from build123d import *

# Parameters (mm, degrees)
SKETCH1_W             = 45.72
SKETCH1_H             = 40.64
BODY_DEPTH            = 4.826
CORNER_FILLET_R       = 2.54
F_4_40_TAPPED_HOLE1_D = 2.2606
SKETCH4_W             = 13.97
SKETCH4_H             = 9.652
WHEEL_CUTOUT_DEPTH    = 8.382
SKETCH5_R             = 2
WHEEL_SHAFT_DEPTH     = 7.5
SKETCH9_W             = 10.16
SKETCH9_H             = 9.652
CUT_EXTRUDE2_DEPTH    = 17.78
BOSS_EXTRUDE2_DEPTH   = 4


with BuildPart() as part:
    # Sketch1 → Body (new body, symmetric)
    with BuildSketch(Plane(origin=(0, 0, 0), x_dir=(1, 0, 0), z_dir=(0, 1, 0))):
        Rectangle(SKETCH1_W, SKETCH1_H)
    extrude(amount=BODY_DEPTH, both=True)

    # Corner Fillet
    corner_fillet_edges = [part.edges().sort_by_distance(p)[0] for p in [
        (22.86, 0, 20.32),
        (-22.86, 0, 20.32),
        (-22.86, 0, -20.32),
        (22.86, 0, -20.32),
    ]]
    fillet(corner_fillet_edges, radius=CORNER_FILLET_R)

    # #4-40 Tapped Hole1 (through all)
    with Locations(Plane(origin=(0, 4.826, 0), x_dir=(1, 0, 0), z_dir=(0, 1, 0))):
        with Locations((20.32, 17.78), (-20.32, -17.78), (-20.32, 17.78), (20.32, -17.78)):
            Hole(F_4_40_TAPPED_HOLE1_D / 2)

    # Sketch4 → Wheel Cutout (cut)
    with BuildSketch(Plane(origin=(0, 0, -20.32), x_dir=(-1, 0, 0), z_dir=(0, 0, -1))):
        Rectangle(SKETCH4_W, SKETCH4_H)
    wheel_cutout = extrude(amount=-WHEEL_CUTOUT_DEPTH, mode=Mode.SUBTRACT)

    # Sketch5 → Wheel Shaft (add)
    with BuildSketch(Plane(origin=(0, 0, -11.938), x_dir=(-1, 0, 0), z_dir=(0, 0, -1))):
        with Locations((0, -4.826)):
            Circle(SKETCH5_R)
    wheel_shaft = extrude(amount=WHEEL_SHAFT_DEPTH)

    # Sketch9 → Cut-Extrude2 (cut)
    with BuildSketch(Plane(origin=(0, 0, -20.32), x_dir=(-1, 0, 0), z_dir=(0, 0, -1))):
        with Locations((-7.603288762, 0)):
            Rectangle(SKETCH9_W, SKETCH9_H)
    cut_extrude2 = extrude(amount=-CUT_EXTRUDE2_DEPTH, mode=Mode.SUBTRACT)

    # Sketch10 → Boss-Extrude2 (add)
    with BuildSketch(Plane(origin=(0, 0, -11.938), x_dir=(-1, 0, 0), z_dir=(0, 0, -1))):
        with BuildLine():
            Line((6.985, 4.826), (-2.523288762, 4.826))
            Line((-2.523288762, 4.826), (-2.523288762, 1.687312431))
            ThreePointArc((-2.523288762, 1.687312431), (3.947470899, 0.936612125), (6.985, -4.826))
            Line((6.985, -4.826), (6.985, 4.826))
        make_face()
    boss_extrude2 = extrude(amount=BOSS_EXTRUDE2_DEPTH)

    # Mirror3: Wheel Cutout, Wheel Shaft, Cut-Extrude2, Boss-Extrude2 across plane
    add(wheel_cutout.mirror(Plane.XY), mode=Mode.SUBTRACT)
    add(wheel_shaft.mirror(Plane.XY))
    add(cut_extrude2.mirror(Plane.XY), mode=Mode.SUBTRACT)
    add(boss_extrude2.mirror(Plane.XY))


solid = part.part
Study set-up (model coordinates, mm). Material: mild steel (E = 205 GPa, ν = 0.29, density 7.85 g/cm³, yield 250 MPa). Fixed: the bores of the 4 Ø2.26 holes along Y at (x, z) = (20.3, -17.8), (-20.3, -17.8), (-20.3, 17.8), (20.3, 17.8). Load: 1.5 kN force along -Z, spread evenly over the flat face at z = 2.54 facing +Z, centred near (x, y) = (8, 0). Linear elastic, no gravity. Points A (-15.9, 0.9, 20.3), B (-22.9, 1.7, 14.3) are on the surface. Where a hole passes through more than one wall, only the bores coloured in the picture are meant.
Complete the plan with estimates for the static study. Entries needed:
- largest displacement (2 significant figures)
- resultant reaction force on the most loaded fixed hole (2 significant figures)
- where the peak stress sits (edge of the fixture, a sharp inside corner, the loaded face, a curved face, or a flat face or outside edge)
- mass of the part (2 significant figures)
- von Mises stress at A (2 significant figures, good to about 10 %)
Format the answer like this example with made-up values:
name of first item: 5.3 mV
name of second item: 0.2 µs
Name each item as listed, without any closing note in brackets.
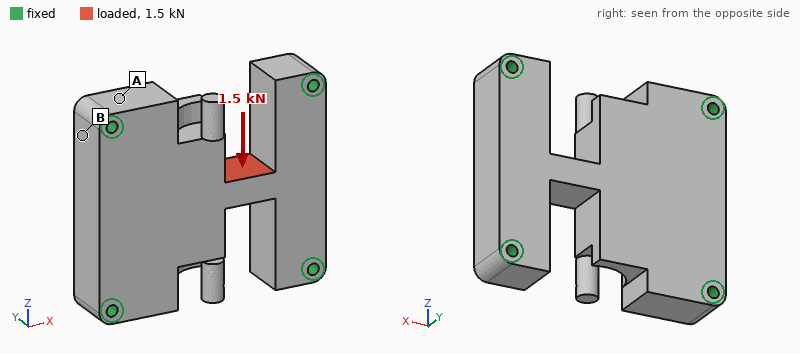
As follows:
largest displacement: 2.3 µm
resultant reaction force on the most loaded fixed hole: 580 N
where the peak stress sits: a flat face or outside edge
mass of the part: 100 g
von Mises stress at A: 4.8 MPa
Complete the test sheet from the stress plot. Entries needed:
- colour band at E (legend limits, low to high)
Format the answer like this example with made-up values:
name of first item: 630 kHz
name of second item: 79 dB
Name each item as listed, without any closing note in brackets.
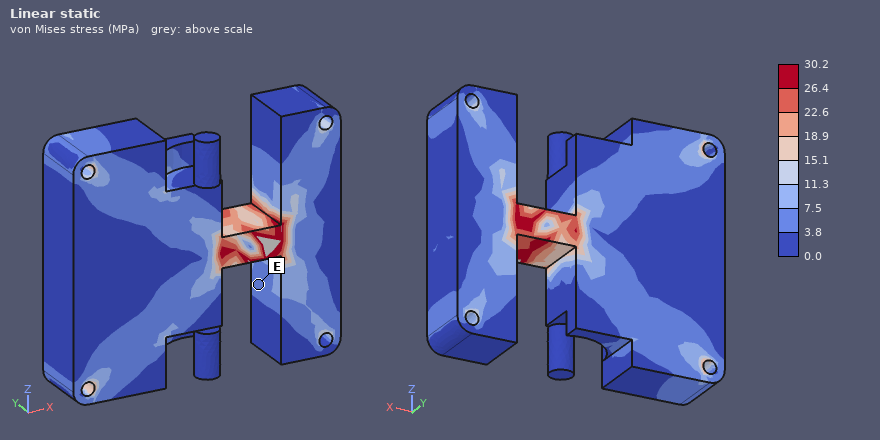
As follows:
colour band at E: 3.8 to 7.5 MPa
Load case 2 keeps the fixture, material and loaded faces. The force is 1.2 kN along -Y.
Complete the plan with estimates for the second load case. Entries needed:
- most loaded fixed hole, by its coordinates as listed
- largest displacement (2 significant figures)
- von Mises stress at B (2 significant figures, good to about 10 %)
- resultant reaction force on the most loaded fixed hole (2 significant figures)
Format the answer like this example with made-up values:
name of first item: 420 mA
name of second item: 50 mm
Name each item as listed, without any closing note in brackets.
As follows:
most loaded fixed hole, by its coordinates as listed: (20.3, 17.8)
largest displacement: 6.8 µm
von Mises stress at B: 11 MPa
resultant reaction force on the most loaded fixed hole: 440 N
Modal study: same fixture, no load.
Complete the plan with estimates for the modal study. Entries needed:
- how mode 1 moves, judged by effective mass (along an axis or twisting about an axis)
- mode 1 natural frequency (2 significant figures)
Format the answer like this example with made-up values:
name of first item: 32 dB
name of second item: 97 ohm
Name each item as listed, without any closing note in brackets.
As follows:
how mode 1 moves, judged by effective mass: along Y
mode 1 natural frequency: 13 kHz
